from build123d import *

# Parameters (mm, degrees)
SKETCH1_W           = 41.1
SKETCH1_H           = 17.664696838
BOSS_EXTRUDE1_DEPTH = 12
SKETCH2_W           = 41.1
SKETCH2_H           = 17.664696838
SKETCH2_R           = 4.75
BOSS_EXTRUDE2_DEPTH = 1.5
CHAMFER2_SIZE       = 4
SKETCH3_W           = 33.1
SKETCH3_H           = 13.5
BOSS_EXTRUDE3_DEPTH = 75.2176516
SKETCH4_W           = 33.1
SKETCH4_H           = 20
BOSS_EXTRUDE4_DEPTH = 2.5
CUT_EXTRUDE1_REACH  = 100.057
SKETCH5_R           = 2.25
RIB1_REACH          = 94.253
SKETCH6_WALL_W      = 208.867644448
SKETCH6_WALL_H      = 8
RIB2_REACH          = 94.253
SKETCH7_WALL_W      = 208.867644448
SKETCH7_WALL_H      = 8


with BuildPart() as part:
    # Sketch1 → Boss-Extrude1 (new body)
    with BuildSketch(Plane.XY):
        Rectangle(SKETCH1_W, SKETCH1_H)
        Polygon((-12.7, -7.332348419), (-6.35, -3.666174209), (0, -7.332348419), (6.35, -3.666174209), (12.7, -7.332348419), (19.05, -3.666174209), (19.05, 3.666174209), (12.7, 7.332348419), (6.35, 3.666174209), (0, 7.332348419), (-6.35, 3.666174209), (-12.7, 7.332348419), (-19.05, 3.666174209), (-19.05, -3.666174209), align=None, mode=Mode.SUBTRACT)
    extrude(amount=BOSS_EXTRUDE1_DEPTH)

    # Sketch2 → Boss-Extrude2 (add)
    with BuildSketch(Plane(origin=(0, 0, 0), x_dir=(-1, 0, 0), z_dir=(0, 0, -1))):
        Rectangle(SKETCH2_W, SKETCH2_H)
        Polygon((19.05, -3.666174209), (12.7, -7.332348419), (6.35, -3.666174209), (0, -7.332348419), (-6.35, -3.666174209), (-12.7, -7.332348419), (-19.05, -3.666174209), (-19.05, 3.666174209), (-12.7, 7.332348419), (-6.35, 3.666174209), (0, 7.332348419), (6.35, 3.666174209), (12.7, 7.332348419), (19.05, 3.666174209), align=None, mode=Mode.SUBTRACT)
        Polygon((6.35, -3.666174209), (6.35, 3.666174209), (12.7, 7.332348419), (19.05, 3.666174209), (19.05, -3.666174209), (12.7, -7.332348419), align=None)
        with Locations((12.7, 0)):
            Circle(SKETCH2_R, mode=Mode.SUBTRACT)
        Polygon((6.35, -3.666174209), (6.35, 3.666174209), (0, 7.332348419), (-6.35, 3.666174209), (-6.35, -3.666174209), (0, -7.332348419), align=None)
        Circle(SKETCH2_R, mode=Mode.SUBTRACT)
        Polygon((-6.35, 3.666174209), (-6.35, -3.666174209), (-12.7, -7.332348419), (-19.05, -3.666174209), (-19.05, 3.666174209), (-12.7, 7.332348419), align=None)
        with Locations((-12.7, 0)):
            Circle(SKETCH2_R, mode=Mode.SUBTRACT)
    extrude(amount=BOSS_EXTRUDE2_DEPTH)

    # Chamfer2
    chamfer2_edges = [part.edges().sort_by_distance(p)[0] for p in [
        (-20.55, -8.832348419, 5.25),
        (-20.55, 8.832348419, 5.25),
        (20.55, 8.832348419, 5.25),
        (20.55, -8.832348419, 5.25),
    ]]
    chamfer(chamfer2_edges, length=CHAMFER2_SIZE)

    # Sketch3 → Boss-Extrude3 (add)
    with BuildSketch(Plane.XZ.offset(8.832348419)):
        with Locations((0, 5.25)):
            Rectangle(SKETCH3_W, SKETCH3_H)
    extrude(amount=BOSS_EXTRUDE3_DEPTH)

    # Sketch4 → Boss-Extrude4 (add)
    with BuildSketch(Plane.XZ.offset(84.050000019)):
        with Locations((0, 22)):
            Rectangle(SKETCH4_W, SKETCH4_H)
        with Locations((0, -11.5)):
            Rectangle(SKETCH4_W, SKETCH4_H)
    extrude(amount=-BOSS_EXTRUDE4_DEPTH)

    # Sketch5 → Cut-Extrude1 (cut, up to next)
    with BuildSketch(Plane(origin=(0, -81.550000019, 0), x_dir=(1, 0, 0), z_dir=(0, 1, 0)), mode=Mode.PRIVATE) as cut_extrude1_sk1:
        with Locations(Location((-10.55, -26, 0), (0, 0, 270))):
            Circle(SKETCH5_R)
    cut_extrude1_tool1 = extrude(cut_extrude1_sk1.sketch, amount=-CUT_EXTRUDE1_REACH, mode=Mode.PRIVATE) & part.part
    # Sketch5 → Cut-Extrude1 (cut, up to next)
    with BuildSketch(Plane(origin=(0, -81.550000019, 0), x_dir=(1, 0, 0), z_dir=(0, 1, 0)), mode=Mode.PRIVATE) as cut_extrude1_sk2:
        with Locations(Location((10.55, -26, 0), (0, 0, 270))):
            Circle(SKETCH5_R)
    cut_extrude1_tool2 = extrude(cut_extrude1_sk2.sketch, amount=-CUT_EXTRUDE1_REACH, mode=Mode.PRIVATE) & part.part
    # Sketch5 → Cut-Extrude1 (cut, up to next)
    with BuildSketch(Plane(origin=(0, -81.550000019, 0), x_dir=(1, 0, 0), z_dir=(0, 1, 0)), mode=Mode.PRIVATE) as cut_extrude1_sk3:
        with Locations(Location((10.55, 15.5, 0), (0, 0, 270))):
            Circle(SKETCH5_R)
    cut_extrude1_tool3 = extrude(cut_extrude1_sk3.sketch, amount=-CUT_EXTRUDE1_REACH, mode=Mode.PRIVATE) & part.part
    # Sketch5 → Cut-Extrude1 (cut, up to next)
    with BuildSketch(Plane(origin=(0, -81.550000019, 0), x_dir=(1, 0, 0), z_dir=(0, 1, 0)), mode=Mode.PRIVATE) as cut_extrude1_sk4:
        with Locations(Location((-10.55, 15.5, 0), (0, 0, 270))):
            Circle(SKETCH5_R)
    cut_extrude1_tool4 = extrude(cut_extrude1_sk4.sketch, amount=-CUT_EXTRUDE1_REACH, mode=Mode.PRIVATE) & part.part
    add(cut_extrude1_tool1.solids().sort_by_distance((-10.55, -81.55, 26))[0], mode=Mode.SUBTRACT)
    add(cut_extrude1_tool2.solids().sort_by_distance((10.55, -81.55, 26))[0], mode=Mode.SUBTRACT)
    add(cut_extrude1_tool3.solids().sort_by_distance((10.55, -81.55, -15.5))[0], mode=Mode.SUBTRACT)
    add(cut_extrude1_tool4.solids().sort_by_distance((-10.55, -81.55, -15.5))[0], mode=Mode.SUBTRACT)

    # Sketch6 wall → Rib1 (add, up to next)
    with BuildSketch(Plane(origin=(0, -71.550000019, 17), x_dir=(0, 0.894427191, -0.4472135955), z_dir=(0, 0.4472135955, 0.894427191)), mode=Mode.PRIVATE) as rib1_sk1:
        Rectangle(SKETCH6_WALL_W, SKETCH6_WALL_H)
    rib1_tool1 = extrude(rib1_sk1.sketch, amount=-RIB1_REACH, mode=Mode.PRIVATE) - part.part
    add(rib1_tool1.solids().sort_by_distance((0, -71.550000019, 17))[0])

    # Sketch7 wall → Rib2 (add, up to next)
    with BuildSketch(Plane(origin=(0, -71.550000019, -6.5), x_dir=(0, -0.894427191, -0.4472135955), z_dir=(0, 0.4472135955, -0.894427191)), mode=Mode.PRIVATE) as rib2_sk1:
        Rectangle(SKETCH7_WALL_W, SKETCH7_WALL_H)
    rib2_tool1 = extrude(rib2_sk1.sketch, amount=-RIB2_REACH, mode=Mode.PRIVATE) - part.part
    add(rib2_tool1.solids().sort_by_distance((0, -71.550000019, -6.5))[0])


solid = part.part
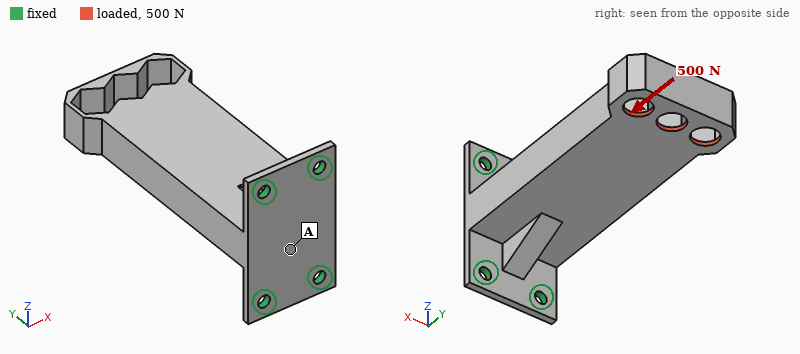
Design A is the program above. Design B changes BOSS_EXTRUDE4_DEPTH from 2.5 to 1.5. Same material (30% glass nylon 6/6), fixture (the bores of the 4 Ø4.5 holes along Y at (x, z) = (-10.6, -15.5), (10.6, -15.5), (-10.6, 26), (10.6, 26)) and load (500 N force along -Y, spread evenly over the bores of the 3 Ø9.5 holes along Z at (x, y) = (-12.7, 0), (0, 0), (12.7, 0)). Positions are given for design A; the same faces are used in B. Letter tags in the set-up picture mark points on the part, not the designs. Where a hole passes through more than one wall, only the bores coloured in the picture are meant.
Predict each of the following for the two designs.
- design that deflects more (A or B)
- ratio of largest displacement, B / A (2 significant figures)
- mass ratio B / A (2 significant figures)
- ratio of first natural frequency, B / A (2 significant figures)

B
1.7
0.97
0.57
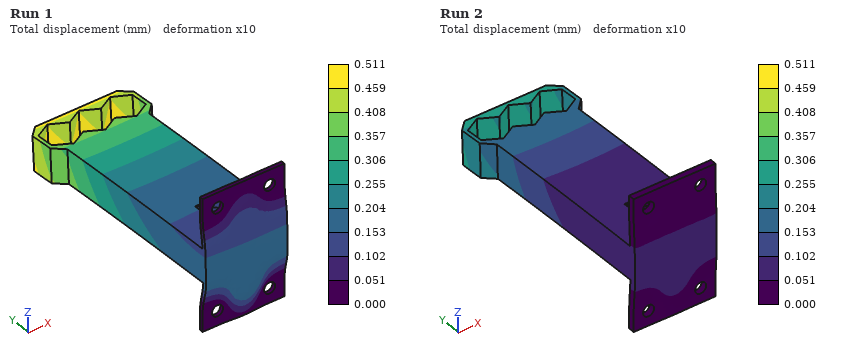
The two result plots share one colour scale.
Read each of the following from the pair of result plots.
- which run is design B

Run 1
